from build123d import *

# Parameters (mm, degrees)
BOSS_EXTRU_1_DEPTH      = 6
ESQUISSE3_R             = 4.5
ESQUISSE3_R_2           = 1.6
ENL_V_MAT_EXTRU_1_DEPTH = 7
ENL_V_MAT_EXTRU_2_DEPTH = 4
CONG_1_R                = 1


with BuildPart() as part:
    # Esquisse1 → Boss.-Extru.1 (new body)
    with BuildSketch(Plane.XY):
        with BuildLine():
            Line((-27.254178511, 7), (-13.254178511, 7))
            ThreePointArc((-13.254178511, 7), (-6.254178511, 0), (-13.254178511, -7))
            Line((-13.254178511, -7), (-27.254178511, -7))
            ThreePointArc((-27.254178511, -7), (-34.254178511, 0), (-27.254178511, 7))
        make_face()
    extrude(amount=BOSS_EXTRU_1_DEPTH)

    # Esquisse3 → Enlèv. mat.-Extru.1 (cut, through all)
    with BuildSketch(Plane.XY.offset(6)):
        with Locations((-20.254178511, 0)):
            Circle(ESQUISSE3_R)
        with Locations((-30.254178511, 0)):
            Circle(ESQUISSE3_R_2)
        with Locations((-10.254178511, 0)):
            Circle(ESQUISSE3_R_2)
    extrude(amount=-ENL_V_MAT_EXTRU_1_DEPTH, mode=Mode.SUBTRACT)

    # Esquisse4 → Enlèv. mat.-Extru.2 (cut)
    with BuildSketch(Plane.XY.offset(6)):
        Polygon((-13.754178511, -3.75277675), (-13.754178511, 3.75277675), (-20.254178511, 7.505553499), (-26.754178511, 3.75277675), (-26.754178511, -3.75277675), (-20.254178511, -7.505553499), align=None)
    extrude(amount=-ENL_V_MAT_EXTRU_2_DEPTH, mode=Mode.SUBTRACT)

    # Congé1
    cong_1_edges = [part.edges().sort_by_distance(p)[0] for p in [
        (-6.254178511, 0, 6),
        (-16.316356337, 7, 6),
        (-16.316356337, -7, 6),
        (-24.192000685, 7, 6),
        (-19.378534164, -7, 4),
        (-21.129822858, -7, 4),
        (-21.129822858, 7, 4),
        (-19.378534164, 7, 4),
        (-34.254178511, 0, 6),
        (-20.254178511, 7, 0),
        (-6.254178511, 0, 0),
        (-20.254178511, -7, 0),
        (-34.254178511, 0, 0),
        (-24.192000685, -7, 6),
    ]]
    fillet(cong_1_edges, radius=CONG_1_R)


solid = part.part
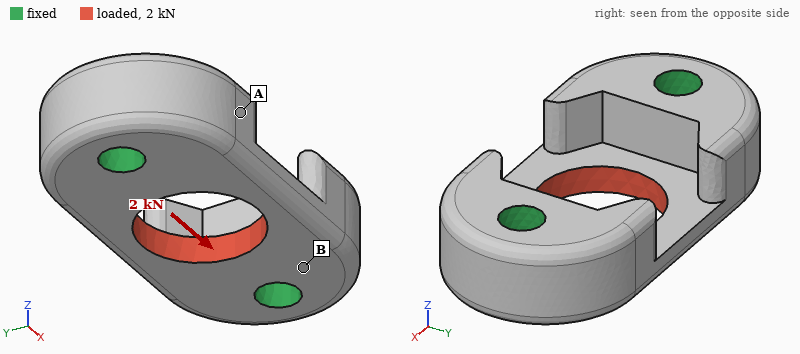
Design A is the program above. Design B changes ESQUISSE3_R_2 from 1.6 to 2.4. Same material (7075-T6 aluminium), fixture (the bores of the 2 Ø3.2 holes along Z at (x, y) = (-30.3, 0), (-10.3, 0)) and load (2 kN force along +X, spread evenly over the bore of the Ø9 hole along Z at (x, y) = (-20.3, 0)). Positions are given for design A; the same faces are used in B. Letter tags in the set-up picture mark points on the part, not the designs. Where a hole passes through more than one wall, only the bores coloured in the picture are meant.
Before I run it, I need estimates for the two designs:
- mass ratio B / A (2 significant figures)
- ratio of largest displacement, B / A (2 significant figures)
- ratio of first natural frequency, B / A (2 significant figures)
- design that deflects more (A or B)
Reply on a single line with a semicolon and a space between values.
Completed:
0.90; 0.88; 1.1; A
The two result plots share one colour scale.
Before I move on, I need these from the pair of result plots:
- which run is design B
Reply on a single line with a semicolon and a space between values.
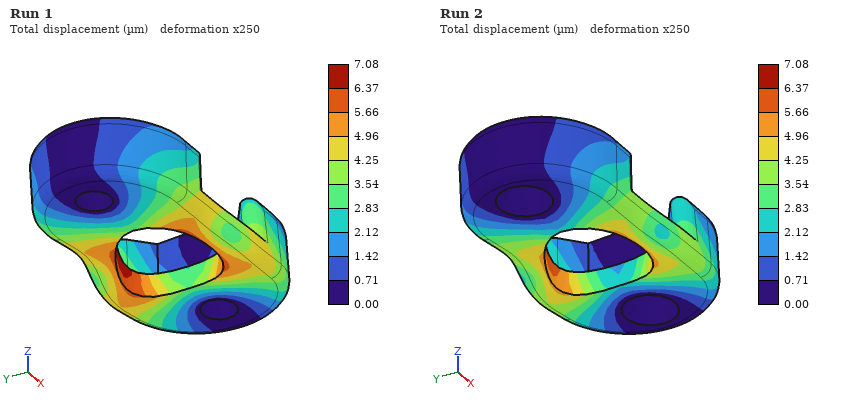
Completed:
Run 2
